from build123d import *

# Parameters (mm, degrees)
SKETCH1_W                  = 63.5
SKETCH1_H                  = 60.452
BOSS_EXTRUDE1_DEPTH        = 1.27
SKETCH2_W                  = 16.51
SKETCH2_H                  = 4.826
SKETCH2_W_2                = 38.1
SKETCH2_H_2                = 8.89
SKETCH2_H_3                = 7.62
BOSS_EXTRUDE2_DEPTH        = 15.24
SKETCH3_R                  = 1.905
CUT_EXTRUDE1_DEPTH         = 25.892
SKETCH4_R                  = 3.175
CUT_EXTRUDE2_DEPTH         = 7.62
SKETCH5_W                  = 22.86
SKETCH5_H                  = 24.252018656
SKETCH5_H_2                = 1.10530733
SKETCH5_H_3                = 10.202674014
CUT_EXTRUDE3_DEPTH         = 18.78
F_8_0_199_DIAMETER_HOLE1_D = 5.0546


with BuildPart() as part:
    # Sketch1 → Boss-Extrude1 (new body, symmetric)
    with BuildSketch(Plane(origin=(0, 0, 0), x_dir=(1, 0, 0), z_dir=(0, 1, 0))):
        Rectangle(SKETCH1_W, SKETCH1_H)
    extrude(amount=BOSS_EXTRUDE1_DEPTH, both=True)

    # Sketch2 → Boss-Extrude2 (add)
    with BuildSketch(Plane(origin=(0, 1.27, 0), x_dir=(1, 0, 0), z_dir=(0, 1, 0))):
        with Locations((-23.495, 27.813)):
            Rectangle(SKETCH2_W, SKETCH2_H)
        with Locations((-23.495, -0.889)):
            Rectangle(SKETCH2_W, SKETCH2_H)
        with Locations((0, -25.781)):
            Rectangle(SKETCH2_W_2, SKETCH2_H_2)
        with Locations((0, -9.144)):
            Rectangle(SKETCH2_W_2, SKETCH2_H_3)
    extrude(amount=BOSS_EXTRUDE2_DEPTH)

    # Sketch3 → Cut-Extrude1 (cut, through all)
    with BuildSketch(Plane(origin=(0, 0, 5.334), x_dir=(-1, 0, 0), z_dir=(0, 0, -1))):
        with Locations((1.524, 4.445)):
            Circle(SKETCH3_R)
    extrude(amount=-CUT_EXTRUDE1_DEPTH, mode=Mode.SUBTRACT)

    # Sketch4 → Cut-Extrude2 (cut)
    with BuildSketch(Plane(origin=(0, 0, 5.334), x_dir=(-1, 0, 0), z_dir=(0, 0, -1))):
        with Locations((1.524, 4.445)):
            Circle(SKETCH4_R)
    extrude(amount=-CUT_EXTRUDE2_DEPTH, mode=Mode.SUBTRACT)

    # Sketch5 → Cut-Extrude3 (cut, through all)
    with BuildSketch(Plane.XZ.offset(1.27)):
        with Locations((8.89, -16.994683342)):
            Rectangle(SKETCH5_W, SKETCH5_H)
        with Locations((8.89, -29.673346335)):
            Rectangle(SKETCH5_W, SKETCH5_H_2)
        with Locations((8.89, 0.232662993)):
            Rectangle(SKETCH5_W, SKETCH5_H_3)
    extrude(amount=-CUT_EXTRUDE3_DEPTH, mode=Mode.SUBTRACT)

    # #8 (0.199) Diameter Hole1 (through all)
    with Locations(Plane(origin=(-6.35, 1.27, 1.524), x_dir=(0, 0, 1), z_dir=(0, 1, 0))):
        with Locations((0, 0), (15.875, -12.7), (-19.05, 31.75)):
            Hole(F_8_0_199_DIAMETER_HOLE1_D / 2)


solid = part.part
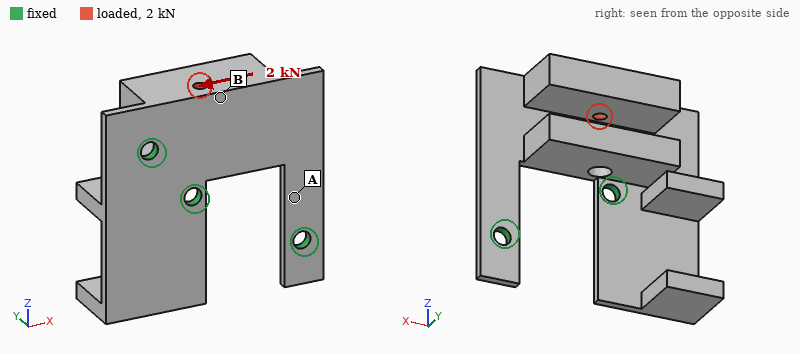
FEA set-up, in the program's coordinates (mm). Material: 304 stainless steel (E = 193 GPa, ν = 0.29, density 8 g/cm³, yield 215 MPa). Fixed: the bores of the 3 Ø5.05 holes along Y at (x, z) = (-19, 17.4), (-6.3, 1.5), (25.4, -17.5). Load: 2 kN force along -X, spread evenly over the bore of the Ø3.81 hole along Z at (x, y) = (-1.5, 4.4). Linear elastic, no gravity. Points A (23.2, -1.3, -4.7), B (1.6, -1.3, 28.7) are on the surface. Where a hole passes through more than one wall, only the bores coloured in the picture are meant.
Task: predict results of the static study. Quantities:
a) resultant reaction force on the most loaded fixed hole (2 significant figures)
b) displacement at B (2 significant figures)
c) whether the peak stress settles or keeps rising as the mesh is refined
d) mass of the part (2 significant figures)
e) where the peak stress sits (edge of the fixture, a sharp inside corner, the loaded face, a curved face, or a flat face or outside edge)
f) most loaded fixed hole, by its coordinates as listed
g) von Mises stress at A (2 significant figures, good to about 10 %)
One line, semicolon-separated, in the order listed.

1.8 kN; 35 µm; keeps rising; 150 g; edge of the fixture; (-19, 17.4); 32 MPa
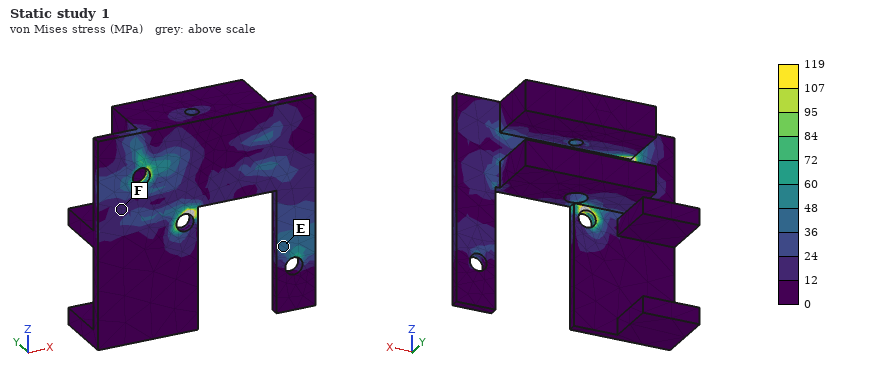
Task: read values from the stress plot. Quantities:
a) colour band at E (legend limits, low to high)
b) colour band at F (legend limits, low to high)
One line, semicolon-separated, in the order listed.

36 to 48 MPa; 12 to 24 MPa
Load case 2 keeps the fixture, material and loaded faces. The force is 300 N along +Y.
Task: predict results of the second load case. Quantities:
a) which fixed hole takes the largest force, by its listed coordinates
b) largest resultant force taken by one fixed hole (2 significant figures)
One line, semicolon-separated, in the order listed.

(-19, 17.4); 240 N
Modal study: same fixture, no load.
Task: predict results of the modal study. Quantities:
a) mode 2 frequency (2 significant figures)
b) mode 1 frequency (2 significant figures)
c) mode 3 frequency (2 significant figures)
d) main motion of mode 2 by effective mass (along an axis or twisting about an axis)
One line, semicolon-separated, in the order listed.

1600 Hz; 1000 Hz; 2600 Hz; along Y
